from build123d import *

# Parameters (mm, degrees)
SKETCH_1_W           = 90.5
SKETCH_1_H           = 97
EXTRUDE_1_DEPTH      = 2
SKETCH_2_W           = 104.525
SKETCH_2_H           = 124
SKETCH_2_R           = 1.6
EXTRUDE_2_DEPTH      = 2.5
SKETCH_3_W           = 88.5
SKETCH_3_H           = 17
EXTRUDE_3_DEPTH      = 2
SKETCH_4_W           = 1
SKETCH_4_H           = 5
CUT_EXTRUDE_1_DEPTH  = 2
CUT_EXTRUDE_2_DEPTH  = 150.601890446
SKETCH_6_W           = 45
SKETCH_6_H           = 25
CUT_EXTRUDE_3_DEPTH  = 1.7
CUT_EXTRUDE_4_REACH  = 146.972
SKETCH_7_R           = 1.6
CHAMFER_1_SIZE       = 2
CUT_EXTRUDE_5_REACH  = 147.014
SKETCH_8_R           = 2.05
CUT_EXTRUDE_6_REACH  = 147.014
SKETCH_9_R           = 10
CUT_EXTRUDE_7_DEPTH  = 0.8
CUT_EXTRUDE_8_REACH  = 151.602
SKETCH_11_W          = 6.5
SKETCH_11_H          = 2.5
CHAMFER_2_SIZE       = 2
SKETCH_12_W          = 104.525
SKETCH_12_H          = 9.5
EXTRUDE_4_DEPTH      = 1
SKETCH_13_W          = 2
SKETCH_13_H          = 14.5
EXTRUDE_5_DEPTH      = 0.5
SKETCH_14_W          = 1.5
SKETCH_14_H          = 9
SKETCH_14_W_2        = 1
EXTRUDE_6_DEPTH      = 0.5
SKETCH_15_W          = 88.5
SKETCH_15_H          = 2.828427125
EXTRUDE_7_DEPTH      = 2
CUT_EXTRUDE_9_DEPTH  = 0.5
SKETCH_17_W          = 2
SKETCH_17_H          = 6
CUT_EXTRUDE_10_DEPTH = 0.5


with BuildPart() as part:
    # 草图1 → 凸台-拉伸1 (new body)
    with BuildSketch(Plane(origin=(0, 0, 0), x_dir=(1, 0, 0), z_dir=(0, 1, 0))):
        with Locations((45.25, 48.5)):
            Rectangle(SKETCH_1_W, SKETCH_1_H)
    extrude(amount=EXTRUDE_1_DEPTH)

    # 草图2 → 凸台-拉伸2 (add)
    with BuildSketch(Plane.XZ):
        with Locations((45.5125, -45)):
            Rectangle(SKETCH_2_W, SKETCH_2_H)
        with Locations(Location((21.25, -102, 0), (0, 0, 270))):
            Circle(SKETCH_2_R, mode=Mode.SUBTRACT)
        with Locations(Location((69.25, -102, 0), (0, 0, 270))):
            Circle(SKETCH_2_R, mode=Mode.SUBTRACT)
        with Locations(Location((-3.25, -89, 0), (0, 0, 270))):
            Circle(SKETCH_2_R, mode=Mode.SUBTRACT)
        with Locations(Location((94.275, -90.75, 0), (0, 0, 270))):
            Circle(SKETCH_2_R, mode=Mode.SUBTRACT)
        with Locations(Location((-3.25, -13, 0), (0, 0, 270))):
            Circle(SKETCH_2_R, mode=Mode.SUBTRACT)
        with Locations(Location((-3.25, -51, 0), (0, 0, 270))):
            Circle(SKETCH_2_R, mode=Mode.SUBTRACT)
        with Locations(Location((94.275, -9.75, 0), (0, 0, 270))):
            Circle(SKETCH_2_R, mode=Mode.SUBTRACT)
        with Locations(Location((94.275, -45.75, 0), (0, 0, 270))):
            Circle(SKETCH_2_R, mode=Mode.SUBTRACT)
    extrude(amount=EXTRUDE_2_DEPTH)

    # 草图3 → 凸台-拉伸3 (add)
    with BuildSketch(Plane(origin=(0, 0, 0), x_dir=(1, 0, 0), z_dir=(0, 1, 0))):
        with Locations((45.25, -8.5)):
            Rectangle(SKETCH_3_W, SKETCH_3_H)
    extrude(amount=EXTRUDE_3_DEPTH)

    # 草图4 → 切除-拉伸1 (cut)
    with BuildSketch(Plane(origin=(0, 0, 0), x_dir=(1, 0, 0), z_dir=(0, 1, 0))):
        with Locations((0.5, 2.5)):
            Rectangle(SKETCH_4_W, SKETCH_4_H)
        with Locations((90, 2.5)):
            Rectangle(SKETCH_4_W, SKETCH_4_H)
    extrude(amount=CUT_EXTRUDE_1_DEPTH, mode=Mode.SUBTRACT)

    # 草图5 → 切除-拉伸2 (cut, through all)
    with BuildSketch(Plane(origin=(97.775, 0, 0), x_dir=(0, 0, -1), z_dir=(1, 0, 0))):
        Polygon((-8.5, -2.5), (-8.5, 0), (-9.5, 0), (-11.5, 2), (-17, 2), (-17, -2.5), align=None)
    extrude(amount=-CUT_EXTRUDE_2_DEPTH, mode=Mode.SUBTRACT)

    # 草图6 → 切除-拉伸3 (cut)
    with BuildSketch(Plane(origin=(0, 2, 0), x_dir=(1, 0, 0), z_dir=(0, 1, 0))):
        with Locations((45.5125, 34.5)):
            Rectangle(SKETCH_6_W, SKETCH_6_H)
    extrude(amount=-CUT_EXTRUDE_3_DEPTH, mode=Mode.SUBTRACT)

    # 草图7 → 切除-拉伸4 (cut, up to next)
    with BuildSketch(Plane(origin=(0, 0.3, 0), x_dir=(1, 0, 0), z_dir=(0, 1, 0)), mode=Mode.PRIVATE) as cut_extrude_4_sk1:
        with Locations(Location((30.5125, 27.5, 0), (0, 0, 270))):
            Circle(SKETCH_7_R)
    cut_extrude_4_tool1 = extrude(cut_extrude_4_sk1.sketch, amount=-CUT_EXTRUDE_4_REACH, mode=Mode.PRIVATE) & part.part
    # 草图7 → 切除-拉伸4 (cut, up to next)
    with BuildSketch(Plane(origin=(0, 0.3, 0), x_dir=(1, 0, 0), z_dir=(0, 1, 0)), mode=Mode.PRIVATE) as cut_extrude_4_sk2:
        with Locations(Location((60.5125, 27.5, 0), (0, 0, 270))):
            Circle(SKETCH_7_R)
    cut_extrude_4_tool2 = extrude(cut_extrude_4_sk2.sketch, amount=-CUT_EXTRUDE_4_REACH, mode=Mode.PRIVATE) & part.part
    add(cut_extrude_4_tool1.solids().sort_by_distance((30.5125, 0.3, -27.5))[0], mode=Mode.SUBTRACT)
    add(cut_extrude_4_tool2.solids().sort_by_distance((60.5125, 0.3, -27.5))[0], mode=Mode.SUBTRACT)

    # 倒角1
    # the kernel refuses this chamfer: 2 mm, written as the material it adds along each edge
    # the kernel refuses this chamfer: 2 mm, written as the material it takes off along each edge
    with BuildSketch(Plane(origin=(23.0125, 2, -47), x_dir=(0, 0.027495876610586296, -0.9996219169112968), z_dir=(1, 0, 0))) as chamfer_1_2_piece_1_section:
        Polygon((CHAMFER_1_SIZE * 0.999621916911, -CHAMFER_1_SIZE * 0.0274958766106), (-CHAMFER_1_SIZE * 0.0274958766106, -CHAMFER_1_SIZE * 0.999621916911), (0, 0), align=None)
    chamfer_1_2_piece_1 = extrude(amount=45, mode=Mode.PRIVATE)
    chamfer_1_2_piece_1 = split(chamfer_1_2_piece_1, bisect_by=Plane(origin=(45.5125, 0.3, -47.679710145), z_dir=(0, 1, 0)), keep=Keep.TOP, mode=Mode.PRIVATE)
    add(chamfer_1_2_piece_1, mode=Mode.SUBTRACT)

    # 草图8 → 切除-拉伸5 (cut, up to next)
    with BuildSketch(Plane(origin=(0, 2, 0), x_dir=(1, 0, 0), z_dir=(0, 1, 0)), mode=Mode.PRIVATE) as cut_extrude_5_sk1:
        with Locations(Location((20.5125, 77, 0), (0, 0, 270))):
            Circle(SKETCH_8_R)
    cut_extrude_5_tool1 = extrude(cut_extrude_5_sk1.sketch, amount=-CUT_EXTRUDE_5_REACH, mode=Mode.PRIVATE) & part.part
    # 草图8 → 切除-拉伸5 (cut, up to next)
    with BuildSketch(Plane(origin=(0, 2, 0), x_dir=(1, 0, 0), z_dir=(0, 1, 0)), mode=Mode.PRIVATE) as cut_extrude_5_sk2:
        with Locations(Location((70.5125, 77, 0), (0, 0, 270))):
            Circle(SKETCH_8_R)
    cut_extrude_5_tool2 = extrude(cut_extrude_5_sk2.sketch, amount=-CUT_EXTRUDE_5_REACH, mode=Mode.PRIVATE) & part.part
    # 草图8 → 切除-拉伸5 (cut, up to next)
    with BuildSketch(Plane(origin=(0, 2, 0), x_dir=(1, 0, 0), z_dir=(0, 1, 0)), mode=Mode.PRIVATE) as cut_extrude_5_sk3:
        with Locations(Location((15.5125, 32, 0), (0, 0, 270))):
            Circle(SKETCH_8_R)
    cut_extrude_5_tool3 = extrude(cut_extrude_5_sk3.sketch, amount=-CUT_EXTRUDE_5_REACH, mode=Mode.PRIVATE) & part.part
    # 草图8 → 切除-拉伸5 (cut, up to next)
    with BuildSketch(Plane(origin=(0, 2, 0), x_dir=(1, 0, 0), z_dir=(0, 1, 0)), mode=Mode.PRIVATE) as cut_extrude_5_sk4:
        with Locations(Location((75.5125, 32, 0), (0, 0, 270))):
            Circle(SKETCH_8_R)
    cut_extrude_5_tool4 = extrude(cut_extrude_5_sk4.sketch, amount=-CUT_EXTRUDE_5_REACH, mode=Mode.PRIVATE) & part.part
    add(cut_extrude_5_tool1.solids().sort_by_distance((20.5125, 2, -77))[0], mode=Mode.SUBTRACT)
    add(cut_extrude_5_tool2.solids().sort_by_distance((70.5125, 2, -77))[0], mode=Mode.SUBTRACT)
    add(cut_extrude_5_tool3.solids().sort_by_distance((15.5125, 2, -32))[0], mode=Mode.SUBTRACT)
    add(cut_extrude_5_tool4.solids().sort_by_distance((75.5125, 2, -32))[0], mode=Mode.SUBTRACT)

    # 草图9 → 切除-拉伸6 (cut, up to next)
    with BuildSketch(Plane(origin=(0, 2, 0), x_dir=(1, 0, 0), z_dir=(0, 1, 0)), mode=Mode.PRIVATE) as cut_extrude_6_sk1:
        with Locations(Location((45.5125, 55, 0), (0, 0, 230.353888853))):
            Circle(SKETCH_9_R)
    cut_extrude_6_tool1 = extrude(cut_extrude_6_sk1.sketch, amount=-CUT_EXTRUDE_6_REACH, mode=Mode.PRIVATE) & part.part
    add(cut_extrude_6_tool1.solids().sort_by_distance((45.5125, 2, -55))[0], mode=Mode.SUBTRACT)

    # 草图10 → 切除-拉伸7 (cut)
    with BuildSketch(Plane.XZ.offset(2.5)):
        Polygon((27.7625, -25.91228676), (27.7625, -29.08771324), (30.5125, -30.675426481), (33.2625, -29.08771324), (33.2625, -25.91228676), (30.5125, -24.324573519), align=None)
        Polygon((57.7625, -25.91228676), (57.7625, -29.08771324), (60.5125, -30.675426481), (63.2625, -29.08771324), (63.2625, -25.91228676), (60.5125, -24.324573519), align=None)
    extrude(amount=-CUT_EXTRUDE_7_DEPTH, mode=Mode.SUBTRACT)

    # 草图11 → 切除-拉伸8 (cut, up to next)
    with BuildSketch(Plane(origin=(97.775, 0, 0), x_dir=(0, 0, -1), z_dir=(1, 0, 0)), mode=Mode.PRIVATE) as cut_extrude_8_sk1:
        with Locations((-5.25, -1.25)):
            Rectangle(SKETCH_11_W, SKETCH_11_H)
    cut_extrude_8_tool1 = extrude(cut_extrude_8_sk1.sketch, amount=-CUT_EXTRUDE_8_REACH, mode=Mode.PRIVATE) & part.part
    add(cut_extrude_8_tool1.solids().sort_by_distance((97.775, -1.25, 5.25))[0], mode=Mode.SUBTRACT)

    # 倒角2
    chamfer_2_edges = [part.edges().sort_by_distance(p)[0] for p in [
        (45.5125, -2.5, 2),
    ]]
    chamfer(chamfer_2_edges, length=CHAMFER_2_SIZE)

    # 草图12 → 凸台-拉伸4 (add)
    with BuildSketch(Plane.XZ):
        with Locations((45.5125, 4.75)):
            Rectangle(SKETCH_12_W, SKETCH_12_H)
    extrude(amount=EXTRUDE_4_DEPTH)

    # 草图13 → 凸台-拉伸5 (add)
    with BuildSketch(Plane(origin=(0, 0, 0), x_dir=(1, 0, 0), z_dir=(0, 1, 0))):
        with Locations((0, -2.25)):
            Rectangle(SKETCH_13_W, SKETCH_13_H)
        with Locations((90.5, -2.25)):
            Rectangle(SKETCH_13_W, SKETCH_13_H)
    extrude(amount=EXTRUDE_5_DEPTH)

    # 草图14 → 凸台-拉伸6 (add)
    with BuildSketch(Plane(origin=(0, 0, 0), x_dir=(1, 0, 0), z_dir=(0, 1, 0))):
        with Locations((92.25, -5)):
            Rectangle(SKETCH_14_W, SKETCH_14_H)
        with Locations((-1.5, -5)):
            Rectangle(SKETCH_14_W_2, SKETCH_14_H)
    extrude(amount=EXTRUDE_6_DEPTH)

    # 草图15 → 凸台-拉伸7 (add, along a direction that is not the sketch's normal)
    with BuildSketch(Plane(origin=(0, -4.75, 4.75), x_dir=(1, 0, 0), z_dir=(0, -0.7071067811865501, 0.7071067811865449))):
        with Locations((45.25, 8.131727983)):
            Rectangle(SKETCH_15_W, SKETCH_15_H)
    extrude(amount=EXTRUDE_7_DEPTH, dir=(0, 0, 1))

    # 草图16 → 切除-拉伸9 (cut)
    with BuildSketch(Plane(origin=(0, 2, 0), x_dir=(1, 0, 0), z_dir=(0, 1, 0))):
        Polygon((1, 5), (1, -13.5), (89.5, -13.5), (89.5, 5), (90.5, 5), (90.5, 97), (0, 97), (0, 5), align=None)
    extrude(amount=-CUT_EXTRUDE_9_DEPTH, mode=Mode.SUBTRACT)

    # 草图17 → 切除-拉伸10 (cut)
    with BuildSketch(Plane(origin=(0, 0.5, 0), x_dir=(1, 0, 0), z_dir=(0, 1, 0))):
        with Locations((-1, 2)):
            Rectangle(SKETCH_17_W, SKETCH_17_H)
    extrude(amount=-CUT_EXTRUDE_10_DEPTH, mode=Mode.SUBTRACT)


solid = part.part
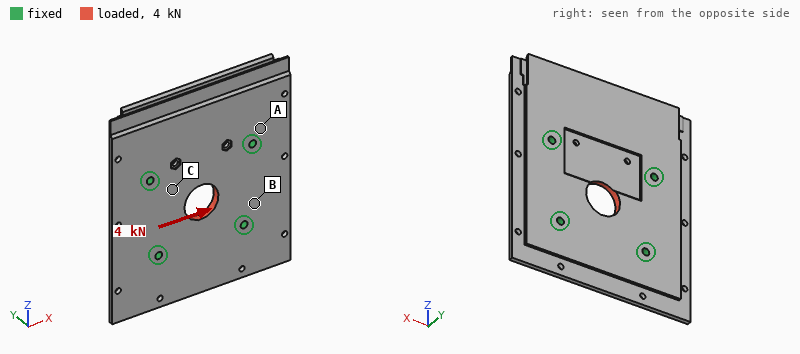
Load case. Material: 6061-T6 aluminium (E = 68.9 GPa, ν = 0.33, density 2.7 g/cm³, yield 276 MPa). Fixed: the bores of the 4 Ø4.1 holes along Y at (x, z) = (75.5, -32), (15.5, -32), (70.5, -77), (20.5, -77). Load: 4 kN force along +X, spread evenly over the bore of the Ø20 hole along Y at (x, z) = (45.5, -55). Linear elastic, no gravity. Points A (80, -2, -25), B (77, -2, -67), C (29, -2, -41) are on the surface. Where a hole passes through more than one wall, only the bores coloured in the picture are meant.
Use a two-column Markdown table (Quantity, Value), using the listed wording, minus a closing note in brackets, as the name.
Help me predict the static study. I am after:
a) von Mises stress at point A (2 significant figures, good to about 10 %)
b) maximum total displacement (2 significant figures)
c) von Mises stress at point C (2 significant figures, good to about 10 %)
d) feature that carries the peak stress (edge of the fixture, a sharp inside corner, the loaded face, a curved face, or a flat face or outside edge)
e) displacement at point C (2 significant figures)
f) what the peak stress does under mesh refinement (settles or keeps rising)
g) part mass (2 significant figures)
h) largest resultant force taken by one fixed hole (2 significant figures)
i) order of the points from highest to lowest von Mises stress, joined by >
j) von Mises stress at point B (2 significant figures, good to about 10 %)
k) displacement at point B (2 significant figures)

| Quantity | Value |
|---|---|
| von Mises stress at point A | 3.4 MPa |
| maximum total displacement | 7.8 µm |
| von Mises stress at point C | 13 MPa |
| feature that carries the peak stress | edge of the fixture |
| displacement at point C | 4.1 µm |
| what the peak stress does under mesh refinement | keeps rising |
| part mass | 110 g |
| largest resultant force taken by one fixed hole | 1.1 kN |
| order of the points from highest to lowest von Mises stress, joined by > | C > B > A |
| von Mises stress at point B | 8.3 MPa |
| displacement at point B | 3.1 µm |
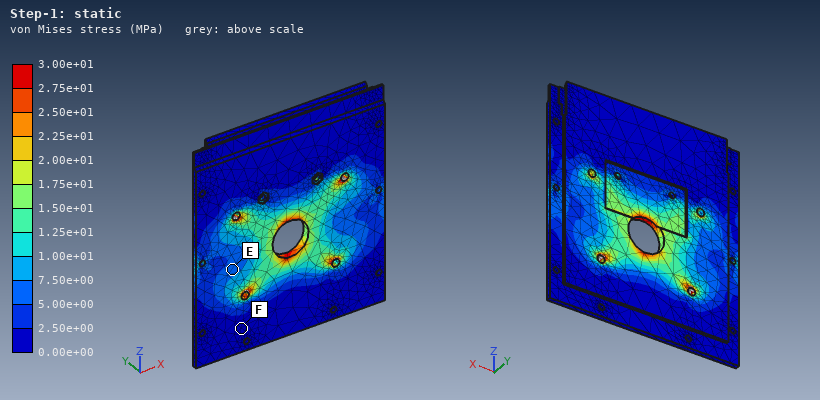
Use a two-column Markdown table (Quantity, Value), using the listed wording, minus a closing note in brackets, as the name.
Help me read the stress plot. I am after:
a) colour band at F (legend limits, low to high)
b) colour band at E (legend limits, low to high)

| Quantity | Value |
|---|---|
| colour band at F | 0.00e+00 to 2.50e+00 MPa |
| colour band at E | 5.00e+00 to 7.50e+00 MPa |
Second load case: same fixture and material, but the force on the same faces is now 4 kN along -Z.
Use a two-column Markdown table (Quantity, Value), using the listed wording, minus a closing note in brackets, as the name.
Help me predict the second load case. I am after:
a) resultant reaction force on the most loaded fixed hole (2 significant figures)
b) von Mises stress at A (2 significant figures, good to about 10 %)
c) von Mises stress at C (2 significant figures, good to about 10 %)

| Quantity | Value |
|---|---|
| resultant reaction force on the most loaded fixed hole | 1.2 kN |
| von Mises stress at A | 5.2 MPa |
| von Mises stress at C | 12 MPa |
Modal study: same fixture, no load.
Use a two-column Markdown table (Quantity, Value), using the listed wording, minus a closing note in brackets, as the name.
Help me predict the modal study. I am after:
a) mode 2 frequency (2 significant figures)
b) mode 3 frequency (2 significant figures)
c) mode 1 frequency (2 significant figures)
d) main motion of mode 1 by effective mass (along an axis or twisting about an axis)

| Quantity | Value |
|---|---|
| mode 2 frequency | 2400 Hz |
| mode 3 frequency | 3300 Hz |
| mode 1 frequency | 1600 Hz |
| main motion of mode 1 by effective mass | along Y |
